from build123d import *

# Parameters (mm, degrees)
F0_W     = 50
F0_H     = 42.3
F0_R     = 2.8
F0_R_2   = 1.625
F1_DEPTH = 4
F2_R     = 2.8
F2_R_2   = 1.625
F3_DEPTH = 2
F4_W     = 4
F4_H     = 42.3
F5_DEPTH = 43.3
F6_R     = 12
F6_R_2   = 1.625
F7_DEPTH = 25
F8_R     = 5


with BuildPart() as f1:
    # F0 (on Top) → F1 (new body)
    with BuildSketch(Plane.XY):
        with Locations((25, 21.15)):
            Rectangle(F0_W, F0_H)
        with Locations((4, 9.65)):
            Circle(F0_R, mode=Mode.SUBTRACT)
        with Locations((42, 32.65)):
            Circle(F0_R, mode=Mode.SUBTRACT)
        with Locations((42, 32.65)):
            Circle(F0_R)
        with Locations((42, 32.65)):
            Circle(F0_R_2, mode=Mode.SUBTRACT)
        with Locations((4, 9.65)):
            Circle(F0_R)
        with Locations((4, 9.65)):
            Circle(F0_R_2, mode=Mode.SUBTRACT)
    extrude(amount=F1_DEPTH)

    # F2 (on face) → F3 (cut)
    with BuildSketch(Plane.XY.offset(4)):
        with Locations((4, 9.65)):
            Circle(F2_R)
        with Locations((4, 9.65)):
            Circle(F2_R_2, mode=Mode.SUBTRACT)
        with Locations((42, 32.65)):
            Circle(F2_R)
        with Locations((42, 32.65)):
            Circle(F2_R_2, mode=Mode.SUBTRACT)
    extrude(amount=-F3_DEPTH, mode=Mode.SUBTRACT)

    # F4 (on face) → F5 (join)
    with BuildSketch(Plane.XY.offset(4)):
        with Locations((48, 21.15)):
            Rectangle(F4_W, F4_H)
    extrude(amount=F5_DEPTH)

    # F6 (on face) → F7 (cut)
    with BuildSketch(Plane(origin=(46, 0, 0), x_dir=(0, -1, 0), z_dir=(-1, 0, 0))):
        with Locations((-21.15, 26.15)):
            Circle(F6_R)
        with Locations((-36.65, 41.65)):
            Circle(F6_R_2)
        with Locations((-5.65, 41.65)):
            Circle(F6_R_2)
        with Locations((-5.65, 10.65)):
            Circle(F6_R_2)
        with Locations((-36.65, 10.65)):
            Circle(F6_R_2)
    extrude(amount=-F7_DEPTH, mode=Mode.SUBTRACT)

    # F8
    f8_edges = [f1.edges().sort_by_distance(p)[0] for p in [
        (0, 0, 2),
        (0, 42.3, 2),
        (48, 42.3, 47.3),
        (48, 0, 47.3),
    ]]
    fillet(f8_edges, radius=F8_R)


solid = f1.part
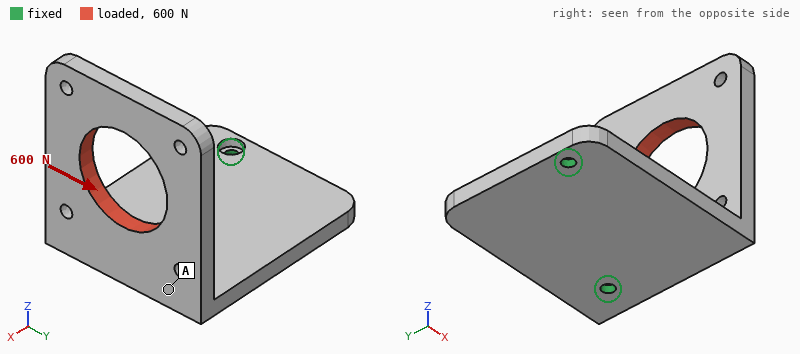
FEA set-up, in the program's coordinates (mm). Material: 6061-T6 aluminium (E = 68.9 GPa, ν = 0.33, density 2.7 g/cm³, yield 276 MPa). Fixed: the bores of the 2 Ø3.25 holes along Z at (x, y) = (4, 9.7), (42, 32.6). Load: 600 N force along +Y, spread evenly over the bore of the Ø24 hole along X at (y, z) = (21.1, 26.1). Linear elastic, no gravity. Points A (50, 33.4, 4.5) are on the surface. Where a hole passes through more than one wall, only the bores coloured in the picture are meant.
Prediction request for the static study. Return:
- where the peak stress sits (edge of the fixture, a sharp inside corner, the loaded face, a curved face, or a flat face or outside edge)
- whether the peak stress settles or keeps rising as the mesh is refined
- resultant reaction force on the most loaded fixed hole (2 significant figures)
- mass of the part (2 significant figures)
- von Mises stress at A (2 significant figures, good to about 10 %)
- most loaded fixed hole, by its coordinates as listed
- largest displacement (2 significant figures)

edge of the fixture
keeps rising
620 N
37 g
39 MPa
(42, 32.6)
0.80 mm
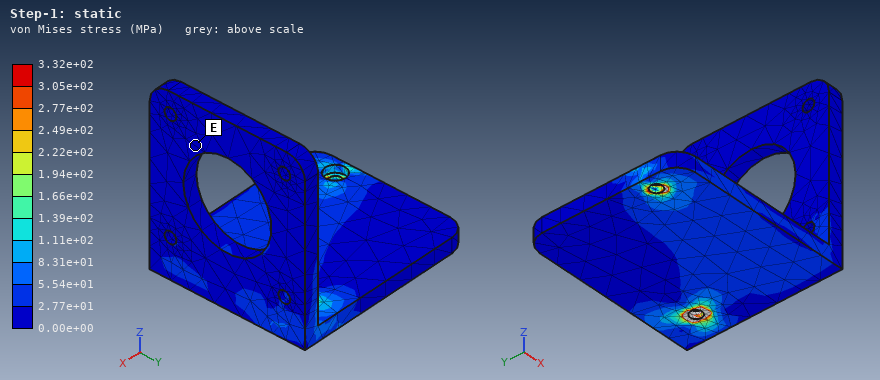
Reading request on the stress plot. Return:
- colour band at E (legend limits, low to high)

0.00e+00 to 2.77e+01 MPa
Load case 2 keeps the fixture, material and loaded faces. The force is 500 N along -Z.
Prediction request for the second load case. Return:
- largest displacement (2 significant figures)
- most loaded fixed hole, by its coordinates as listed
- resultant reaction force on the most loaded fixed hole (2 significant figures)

0.37 mm
(42, 32.6)
490 N
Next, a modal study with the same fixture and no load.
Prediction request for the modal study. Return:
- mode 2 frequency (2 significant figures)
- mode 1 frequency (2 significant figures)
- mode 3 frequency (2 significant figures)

1400 Hz
1000 Hz
3100 Hz
